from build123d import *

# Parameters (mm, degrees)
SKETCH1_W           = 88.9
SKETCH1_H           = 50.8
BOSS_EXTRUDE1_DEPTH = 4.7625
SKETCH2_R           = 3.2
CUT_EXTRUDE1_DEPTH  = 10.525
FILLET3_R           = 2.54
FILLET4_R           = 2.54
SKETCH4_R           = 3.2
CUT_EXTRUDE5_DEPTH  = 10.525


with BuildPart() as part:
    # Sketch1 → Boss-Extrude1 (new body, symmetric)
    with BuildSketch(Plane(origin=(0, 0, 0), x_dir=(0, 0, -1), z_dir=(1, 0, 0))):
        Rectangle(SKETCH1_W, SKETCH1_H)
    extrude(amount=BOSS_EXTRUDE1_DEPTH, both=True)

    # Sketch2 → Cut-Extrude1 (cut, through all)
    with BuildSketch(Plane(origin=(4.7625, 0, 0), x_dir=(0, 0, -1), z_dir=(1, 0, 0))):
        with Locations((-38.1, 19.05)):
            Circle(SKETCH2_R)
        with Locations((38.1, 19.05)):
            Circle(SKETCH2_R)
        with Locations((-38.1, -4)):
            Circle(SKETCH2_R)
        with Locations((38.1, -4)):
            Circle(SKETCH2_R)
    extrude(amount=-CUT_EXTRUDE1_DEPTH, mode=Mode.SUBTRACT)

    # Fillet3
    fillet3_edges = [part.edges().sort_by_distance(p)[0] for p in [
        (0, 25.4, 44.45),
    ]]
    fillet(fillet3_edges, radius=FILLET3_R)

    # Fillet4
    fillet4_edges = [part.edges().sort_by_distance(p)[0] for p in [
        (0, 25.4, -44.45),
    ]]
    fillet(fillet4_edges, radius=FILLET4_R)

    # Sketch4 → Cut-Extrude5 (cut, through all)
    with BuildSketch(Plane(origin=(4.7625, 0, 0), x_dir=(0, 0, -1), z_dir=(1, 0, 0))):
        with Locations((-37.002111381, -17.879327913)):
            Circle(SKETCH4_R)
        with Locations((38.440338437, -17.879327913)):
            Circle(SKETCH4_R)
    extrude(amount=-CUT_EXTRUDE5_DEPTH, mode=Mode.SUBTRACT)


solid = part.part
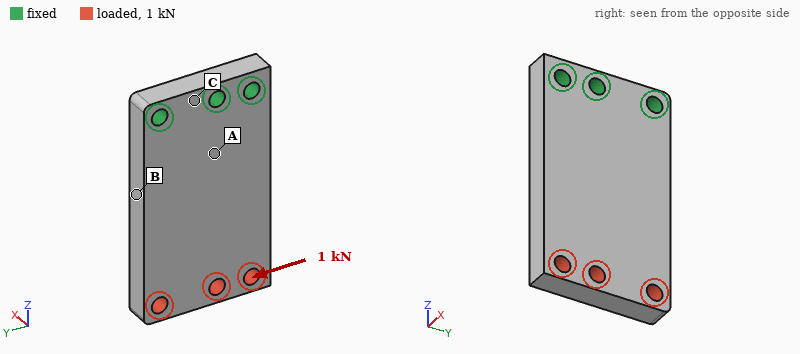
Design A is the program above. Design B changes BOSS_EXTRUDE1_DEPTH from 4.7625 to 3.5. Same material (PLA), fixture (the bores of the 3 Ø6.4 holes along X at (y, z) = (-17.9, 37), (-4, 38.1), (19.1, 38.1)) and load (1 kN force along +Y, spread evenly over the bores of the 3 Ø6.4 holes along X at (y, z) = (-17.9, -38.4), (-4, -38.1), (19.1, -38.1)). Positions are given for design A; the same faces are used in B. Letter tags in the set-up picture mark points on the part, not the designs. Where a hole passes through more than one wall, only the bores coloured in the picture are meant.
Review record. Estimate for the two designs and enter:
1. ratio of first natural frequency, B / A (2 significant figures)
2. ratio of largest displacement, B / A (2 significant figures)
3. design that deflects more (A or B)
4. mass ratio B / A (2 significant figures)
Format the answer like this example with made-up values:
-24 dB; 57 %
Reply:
0.75; 1.4; B; 0.73
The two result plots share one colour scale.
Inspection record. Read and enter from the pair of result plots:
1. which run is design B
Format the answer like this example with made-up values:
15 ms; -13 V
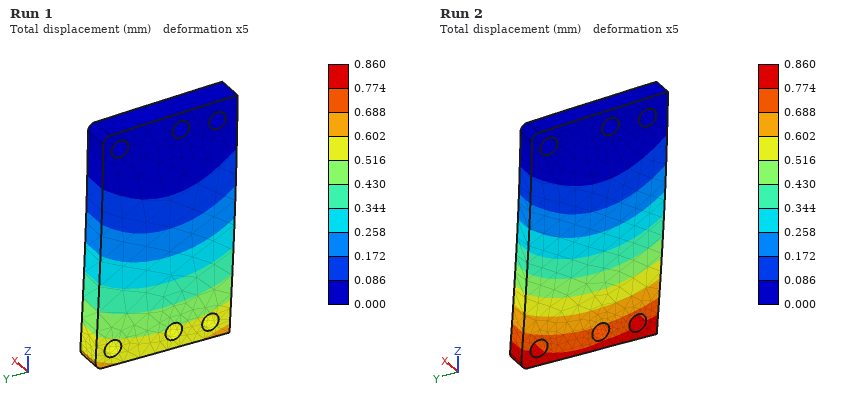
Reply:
Run 2
